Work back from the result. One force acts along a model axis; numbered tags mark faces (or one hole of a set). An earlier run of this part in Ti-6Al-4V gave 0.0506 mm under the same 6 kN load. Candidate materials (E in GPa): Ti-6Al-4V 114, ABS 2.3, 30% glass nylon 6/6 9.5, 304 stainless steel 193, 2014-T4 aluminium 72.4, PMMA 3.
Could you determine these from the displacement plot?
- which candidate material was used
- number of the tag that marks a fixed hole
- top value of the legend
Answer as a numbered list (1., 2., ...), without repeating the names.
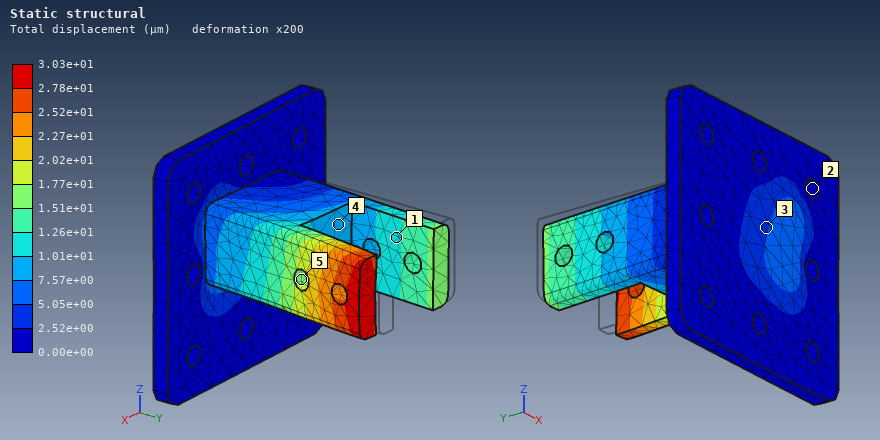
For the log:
1. 304 stainless steel
2. 2
3. 3.03e+01 µm
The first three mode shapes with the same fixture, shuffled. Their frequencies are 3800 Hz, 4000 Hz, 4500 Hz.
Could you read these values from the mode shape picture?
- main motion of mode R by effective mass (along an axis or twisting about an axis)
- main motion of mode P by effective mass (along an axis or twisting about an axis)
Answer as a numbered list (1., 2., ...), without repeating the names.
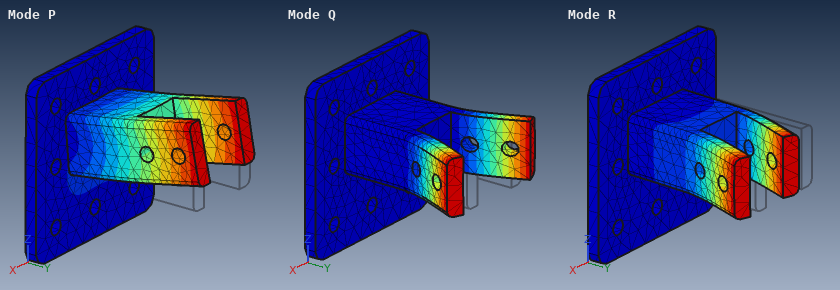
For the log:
1. along X
2. along Z
